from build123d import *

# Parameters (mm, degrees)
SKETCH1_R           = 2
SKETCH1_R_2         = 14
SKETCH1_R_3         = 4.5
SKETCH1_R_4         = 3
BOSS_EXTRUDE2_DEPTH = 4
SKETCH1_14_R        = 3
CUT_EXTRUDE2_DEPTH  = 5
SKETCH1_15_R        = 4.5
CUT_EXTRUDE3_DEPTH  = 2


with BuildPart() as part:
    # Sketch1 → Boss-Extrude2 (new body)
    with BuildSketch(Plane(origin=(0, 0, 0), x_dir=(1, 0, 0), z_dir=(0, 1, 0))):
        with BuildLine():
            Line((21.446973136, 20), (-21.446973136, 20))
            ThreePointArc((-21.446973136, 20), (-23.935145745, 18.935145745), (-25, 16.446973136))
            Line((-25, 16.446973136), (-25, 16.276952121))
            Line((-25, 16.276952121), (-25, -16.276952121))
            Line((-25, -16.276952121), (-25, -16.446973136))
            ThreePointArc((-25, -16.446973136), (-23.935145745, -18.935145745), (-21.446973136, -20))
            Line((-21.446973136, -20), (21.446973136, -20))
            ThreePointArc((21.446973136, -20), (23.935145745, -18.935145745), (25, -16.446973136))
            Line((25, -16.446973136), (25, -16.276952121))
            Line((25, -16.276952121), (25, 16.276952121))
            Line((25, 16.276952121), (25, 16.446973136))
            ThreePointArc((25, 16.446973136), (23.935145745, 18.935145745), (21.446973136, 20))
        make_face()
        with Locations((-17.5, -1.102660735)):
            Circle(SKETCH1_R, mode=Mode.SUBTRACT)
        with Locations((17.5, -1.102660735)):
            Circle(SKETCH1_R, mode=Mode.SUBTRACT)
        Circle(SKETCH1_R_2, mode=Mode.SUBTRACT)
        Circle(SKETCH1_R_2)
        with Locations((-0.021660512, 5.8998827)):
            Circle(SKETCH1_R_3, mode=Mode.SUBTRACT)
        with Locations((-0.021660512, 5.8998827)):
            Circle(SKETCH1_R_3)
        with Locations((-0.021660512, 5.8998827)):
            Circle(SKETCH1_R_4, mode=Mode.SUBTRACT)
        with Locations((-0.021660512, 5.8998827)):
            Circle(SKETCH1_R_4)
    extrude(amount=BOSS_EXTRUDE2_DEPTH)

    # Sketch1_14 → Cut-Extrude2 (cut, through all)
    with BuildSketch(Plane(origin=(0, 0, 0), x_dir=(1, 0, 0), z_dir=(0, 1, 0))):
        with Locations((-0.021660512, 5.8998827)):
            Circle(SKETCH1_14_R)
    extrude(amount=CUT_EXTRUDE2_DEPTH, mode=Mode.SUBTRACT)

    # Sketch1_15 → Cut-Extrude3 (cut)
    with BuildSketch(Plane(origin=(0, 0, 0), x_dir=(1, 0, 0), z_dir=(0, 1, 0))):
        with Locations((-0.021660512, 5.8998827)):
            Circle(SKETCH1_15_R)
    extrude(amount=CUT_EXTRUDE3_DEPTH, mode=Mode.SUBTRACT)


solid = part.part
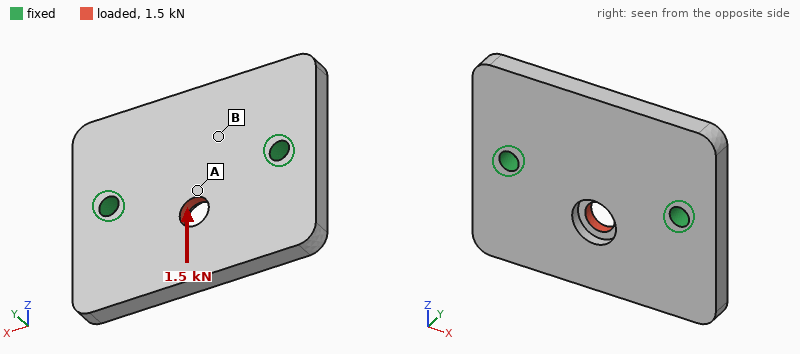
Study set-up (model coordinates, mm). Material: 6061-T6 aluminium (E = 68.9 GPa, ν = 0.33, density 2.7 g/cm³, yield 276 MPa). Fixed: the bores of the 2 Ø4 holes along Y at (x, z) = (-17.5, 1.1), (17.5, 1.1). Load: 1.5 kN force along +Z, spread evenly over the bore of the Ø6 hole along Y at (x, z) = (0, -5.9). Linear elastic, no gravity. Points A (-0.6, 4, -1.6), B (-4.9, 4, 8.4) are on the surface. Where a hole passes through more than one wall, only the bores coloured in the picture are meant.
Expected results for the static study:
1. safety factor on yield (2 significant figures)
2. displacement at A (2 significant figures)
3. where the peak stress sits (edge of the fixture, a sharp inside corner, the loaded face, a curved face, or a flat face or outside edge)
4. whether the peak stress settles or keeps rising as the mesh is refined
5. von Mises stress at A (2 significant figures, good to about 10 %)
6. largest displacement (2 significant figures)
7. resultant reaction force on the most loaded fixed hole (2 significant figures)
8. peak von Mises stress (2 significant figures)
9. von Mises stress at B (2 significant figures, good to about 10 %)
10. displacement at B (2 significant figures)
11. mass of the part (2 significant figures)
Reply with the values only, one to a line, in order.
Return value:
3.8
7.5 µm
the loaded face
settles
37 MPa
18 µm
760 N
72 MPa
9.2 MPa
4.7 µm
21 g
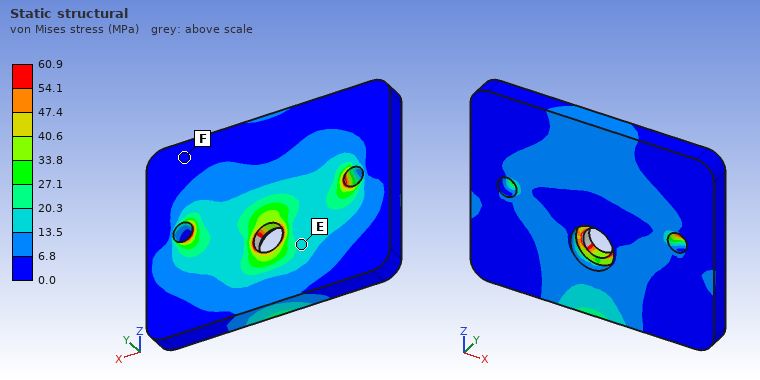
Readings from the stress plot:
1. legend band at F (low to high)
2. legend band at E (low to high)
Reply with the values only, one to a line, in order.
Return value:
0.0 to 6.8 MPa
13.5 to 20.3 MPa
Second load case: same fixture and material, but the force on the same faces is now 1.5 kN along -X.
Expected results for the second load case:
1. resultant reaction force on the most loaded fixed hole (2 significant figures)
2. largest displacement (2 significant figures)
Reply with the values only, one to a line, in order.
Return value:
800 N
7.0 µm
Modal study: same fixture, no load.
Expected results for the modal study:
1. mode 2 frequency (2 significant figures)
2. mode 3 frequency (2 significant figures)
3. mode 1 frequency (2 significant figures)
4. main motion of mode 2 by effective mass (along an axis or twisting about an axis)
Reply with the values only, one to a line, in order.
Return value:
8100 Hz
10000 Hz
6000 Hz
along Y
